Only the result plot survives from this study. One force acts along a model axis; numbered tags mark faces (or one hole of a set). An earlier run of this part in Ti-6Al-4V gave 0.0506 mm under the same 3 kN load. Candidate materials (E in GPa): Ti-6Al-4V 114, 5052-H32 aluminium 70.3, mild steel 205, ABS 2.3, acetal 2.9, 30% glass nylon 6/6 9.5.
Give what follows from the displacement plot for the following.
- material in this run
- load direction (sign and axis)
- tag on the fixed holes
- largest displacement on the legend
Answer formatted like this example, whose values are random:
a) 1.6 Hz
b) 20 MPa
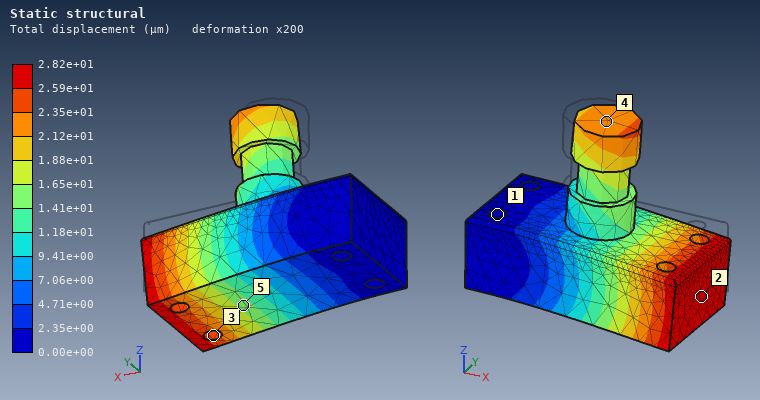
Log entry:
a) mild steel
b) -Z
c) 1
d) 2.82e+01 µm
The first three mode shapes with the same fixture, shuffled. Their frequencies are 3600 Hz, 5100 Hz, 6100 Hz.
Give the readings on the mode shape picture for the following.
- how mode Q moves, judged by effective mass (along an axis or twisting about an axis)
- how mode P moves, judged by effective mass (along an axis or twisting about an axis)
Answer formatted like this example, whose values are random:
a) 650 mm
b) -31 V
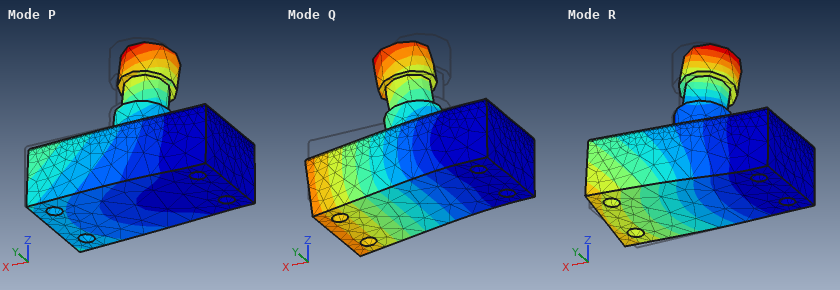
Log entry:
a) along Z
b) along Y
